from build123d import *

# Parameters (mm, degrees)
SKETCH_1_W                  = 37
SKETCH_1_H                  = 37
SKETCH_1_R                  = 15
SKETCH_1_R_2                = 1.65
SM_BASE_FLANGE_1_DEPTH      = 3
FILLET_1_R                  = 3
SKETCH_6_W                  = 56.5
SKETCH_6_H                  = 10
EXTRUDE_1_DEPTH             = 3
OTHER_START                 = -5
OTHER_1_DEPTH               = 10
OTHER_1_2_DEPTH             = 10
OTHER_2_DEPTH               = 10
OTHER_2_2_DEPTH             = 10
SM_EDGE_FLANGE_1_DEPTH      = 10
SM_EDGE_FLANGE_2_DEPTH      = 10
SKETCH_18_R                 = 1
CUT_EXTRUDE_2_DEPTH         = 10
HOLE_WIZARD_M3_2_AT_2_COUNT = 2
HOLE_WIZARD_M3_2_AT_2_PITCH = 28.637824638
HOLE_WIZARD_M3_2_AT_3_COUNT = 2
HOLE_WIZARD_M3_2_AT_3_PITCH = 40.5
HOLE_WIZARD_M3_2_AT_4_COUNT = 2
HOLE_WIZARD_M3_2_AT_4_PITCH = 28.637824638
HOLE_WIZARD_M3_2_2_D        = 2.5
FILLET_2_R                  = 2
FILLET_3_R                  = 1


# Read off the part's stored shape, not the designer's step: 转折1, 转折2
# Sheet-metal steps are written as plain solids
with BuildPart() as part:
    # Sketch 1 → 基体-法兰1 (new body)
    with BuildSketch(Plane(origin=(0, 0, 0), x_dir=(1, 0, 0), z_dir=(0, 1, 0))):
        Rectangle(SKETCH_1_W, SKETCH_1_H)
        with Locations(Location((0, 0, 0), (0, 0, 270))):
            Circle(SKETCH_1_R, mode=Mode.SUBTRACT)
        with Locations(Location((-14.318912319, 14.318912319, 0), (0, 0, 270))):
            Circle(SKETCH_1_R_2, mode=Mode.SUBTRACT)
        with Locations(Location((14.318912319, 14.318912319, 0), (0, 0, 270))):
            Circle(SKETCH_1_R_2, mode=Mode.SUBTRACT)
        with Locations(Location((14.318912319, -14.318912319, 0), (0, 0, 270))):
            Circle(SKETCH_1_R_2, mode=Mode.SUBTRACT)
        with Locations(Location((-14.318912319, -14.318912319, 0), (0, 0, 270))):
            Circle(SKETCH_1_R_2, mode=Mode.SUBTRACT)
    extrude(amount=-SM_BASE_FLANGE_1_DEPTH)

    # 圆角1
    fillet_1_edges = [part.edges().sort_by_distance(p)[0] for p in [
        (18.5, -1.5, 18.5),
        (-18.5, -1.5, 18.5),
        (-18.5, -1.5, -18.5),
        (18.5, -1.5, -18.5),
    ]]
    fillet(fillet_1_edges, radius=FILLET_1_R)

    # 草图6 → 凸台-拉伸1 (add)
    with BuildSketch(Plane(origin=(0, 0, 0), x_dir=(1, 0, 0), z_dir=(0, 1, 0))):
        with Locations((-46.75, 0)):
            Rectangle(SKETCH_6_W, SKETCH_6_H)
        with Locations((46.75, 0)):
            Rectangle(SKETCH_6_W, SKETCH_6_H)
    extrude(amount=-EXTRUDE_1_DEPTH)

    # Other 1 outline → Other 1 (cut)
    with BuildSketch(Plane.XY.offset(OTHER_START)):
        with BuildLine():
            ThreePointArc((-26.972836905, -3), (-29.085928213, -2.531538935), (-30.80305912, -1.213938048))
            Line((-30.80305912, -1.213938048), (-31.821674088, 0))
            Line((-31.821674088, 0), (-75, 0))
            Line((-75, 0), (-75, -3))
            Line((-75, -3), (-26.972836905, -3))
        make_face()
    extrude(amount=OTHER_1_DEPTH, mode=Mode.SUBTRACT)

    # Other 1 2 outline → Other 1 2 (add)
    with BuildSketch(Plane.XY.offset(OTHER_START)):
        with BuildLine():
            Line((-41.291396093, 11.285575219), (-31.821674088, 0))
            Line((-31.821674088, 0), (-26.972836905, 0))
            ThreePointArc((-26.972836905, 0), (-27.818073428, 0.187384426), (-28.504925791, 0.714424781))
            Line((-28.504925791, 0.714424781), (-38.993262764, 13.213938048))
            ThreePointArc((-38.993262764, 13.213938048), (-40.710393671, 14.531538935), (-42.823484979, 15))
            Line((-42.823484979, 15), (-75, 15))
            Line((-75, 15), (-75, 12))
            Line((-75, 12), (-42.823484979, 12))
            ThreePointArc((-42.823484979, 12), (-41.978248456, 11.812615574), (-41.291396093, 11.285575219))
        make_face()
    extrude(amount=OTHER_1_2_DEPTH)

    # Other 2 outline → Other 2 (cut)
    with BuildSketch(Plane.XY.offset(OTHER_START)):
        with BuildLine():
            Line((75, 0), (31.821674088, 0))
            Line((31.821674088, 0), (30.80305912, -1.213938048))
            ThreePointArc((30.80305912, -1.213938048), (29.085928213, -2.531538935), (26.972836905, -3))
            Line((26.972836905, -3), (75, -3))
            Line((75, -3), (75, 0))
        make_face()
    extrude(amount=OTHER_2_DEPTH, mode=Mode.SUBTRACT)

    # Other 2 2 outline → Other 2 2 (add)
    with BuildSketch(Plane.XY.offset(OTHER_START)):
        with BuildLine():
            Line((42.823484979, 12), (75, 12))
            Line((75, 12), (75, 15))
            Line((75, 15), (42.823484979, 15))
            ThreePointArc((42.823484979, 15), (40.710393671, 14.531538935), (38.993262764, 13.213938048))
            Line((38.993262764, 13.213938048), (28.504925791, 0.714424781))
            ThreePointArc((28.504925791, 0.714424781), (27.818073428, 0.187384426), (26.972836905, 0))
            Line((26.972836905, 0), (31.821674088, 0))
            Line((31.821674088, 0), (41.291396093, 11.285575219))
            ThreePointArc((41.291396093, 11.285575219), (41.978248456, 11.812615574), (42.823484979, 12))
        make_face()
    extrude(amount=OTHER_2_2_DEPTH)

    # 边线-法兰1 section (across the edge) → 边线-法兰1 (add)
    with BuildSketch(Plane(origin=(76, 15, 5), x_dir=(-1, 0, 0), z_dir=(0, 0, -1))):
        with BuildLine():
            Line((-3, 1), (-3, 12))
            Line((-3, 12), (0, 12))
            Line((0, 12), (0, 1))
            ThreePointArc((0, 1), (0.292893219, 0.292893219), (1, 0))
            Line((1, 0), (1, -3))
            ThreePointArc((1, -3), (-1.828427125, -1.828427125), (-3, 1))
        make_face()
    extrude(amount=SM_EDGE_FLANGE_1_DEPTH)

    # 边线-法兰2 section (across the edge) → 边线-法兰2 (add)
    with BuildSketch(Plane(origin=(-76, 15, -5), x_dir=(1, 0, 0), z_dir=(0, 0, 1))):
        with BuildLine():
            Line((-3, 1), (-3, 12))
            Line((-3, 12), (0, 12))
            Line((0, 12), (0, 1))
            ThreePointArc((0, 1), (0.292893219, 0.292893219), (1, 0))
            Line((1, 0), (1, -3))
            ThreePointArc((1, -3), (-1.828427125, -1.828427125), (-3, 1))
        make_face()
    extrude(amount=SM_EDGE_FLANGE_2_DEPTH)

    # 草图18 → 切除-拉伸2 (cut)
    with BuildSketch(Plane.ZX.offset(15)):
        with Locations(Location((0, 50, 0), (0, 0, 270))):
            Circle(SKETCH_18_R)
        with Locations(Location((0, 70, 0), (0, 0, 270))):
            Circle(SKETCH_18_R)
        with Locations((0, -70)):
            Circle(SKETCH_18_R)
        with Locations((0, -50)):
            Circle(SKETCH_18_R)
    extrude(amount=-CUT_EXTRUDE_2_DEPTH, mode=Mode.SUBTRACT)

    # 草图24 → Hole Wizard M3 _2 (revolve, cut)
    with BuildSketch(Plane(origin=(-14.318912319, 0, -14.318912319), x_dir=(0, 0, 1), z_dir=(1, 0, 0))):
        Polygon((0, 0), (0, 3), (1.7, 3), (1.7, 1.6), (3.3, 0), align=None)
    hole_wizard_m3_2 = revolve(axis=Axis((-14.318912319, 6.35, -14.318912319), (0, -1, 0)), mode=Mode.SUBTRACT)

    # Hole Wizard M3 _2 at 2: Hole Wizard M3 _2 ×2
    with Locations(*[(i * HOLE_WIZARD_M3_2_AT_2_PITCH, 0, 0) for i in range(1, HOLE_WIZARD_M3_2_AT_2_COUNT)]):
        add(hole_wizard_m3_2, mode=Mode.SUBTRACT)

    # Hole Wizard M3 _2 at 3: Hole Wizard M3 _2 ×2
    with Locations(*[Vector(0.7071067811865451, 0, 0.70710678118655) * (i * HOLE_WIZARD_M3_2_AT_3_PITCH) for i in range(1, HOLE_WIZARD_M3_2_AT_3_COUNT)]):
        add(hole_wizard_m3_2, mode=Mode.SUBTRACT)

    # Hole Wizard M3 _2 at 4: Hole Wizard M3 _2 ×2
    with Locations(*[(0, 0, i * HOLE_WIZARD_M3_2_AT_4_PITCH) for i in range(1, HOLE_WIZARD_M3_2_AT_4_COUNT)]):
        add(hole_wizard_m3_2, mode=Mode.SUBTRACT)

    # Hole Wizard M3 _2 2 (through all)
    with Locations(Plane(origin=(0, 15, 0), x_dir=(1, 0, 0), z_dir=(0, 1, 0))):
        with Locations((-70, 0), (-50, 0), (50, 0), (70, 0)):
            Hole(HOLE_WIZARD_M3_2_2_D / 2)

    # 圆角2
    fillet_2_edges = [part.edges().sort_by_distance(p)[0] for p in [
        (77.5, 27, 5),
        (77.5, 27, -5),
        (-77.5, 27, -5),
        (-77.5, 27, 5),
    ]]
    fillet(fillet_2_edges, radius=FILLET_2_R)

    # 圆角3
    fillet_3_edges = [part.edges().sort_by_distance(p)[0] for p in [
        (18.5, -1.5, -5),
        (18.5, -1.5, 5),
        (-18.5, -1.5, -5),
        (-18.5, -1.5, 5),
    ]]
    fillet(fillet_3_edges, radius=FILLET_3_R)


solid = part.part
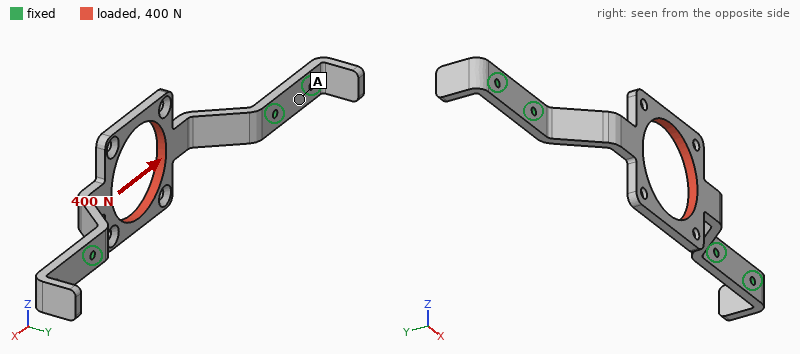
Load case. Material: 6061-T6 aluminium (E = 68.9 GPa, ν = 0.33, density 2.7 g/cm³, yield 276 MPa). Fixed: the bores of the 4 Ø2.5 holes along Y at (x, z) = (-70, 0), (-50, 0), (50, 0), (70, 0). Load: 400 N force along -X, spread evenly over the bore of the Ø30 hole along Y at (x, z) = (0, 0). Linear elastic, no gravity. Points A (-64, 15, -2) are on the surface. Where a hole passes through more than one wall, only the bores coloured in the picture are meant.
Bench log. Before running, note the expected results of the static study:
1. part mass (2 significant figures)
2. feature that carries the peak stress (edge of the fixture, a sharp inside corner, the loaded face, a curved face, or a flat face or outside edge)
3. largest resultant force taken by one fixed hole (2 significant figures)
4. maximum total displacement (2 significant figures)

17 g
a curved face
190 N
0.19 mm
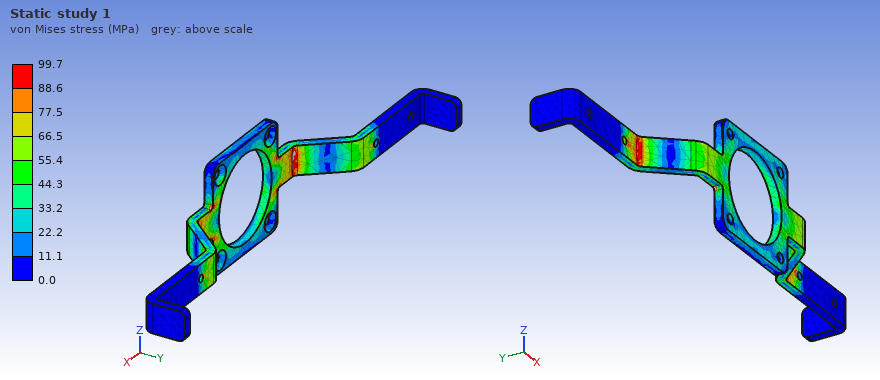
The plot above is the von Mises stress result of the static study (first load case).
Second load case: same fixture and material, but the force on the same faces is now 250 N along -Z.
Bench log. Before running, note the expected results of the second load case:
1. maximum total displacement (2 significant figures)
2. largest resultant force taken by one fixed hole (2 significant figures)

0.25 mm
210 N
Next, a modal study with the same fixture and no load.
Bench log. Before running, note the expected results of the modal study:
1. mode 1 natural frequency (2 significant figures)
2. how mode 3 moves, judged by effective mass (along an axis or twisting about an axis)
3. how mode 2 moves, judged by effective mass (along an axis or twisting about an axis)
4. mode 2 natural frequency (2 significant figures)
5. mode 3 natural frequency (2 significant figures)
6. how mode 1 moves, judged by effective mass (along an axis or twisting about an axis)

1700 Hz
along X
along Y
2200 Hz
2300 Hz
along Z
